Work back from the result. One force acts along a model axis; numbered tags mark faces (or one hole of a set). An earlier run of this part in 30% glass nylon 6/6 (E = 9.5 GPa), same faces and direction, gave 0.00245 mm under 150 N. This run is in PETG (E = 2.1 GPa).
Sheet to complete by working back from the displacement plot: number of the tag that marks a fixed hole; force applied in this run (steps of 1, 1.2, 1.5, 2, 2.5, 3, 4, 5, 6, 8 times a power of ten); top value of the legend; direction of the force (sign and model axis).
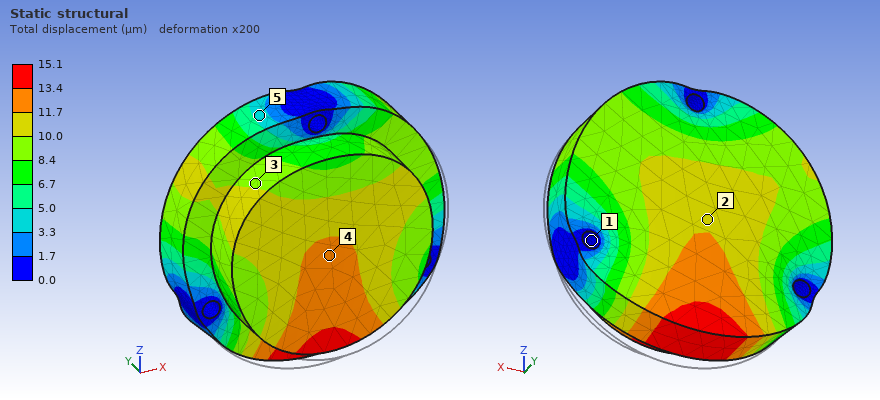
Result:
1
200 N
15.1 µm
+Y
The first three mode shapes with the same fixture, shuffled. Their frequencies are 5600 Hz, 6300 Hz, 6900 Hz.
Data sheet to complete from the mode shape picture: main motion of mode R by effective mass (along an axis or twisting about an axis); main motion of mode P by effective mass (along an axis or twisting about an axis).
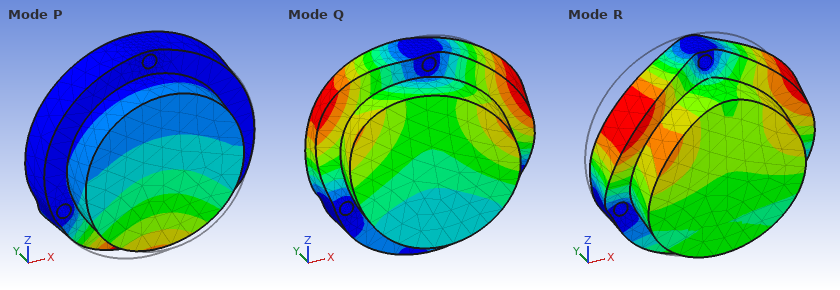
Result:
along Y
along Y
